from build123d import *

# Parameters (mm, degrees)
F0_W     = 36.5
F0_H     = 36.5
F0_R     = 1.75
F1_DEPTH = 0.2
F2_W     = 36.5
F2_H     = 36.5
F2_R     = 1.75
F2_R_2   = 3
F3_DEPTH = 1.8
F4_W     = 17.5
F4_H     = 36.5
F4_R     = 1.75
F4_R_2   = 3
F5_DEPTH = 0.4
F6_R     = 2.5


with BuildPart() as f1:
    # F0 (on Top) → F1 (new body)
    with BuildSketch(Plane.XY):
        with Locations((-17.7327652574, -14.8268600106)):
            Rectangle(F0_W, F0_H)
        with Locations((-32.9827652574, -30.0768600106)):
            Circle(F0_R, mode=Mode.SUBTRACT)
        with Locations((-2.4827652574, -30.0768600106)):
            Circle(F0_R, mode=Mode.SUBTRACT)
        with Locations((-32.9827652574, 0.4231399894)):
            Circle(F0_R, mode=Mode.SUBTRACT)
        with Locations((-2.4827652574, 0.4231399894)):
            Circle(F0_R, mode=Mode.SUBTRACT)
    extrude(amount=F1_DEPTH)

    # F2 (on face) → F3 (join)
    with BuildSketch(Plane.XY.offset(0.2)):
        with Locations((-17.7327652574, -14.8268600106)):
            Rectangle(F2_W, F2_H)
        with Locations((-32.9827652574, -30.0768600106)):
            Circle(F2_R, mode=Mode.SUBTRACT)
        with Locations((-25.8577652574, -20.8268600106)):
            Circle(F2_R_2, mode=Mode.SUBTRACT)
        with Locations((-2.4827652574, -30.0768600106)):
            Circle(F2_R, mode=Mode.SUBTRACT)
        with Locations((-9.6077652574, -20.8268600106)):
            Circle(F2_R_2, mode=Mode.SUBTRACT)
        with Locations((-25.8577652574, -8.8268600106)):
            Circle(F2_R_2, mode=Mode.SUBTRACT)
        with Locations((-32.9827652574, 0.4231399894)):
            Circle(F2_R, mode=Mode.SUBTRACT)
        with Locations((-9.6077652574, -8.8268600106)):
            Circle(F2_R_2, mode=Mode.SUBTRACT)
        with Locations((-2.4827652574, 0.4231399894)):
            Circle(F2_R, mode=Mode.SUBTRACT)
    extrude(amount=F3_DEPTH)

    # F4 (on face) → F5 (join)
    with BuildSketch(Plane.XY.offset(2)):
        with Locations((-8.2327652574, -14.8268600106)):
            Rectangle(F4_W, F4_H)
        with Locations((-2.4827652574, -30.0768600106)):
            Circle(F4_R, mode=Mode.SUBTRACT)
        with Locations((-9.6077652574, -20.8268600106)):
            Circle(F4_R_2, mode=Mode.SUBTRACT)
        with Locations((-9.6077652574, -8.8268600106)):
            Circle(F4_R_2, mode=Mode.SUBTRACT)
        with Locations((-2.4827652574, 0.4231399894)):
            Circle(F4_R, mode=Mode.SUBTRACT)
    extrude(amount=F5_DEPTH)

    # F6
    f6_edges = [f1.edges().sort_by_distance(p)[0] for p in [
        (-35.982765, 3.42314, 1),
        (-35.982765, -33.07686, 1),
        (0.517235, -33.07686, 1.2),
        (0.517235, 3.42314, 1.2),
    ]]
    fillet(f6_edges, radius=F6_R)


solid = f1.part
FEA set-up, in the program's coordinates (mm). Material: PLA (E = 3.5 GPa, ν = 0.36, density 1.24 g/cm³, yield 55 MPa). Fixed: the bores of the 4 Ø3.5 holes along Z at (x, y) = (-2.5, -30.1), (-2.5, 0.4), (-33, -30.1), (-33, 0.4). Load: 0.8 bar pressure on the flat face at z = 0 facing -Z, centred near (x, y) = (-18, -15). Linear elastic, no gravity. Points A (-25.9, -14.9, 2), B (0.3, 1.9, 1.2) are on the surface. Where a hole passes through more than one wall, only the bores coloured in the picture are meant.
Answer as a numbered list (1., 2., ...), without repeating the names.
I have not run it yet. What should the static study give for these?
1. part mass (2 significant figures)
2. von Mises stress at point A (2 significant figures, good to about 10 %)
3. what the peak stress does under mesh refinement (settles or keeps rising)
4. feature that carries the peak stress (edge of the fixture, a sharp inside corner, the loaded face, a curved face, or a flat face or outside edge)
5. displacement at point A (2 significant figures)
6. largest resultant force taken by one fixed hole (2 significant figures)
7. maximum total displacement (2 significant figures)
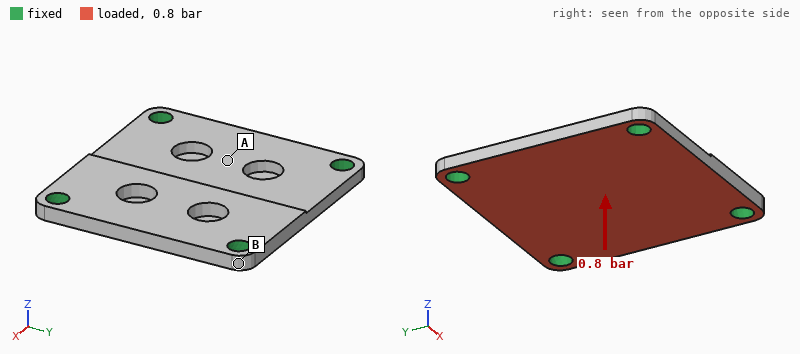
1. 3.2 g
2. 4.0 MPa
3. keeps rising
4. edge of the fixture
5. 0.13 mm
6. 27 N
7. 0.14 mm
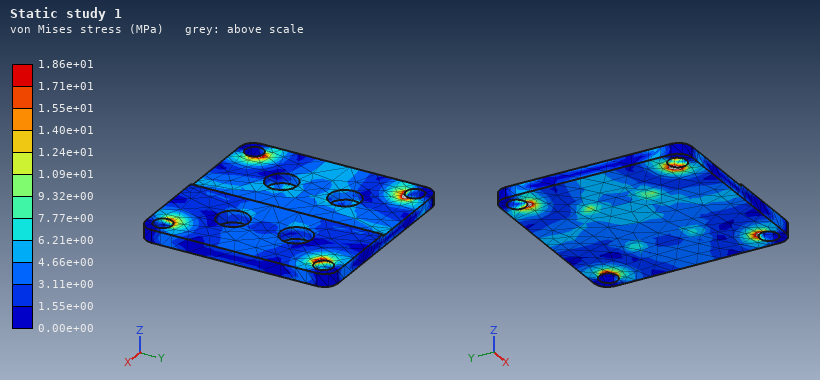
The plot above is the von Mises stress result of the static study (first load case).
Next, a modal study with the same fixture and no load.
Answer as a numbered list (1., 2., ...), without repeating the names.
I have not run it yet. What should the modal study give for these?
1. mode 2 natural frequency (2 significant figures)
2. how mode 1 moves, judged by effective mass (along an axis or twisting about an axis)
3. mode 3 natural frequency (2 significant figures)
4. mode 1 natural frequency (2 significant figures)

1. 4900 Hz
2. along Z
3. 4900 Hz
4. 3000 Hz
